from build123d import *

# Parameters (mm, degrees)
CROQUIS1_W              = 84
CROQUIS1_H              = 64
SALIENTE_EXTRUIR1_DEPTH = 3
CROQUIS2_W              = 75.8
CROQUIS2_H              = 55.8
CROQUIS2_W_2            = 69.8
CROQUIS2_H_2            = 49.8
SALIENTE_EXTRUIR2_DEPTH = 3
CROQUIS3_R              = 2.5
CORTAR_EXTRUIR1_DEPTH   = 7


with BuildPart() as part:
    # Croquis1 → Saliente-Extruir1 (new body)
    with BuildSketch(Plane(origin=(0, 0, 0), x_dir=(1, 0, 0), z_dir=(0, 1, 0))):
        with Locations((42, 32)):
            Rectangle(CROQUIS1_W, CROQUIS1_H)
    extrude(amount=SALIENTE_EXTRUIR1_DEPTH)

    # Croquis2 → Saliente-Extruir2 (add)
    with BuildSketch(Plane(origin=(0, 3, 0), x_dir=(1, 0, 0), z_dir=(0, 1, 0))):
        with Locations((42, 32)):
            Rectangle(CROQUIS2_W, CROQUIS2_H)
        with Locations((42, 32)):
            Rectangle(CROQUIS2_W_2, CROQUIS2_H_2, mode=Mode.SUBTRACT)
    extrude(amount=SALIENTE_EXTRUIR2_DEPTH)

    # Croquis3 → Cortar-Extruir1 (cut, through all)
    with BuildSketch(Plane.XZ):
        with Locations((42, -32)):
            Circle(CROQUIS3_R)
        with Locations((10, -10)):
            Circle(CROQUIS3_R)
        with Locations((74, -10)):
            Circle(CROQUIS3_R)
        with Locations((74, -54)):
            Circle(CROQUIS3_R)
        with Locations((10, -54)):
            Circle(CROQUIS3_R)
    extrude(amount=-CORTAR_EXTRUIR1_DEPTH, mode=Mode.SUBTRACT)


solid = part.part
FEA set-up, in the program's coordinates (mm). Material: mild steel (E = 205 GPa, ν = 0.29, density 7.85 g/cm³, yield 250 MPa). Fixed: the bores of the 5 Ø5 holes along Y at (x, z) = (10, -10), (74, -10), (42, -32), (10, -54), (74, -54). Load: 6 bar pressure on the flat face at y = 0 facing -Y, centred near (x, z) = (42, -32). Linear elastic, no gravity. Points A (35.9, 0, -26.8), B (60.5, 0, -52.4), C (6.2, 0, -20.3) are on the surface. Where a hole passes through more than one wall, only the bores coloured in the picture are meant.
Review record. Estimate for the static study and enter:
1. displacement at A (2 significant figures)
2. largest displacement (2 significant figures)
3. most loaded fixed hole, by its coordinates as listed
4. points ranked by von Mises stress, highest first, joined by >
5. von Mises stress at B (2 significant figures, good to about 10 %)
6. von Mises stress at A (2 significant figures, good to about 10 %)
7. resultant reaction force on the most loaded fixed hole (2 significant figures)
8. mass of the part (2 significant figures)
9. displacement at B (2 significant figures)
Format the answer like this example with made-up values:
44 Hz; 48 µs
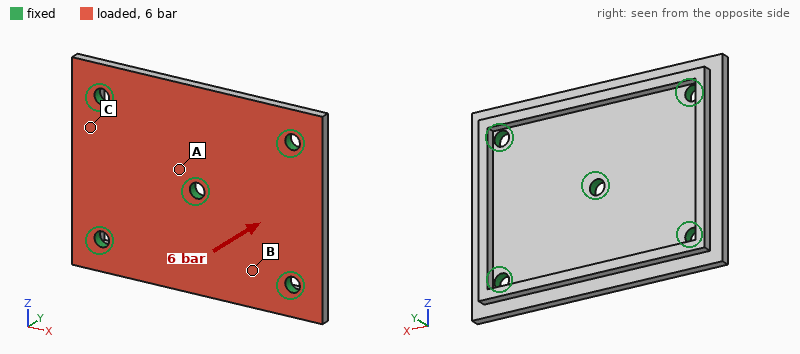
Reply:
3.4 µm; 21 µm; (42, -32); A > B > C; 20 MPa; 28 MPa; 830 N; 140 g; 7.9 µm
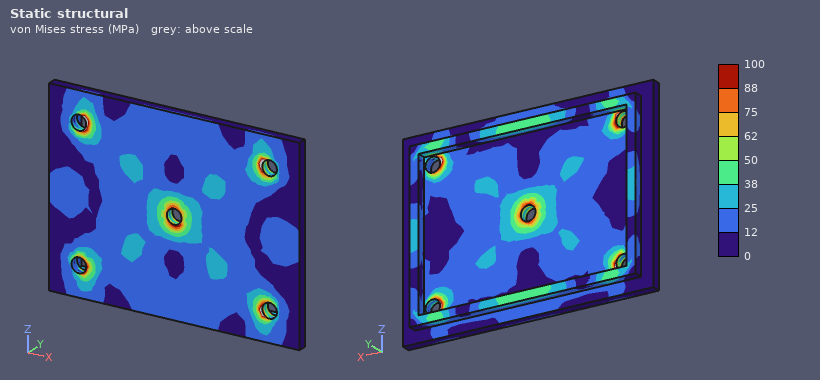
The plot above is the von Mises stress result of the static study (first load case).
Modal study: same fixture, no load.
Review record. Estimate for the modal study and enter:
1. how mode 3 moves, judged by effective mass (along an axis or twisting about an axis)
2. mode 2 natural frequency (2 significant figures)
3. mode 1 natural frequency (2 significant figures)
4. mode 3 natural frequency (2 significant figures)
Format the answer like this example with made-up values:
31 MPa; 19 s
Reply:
twisting about Z; 6400 Hz; 6300 Hz; 10 kHz
